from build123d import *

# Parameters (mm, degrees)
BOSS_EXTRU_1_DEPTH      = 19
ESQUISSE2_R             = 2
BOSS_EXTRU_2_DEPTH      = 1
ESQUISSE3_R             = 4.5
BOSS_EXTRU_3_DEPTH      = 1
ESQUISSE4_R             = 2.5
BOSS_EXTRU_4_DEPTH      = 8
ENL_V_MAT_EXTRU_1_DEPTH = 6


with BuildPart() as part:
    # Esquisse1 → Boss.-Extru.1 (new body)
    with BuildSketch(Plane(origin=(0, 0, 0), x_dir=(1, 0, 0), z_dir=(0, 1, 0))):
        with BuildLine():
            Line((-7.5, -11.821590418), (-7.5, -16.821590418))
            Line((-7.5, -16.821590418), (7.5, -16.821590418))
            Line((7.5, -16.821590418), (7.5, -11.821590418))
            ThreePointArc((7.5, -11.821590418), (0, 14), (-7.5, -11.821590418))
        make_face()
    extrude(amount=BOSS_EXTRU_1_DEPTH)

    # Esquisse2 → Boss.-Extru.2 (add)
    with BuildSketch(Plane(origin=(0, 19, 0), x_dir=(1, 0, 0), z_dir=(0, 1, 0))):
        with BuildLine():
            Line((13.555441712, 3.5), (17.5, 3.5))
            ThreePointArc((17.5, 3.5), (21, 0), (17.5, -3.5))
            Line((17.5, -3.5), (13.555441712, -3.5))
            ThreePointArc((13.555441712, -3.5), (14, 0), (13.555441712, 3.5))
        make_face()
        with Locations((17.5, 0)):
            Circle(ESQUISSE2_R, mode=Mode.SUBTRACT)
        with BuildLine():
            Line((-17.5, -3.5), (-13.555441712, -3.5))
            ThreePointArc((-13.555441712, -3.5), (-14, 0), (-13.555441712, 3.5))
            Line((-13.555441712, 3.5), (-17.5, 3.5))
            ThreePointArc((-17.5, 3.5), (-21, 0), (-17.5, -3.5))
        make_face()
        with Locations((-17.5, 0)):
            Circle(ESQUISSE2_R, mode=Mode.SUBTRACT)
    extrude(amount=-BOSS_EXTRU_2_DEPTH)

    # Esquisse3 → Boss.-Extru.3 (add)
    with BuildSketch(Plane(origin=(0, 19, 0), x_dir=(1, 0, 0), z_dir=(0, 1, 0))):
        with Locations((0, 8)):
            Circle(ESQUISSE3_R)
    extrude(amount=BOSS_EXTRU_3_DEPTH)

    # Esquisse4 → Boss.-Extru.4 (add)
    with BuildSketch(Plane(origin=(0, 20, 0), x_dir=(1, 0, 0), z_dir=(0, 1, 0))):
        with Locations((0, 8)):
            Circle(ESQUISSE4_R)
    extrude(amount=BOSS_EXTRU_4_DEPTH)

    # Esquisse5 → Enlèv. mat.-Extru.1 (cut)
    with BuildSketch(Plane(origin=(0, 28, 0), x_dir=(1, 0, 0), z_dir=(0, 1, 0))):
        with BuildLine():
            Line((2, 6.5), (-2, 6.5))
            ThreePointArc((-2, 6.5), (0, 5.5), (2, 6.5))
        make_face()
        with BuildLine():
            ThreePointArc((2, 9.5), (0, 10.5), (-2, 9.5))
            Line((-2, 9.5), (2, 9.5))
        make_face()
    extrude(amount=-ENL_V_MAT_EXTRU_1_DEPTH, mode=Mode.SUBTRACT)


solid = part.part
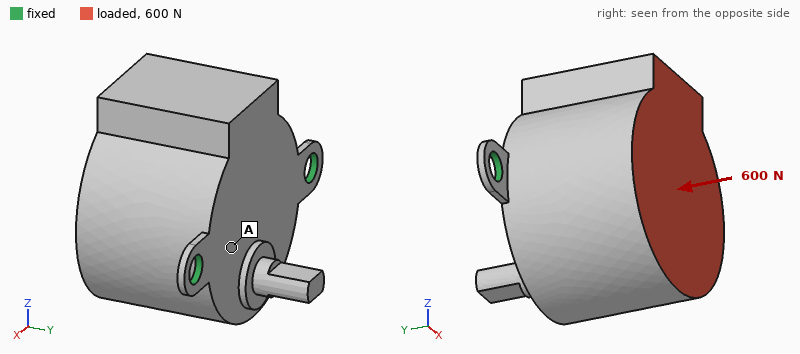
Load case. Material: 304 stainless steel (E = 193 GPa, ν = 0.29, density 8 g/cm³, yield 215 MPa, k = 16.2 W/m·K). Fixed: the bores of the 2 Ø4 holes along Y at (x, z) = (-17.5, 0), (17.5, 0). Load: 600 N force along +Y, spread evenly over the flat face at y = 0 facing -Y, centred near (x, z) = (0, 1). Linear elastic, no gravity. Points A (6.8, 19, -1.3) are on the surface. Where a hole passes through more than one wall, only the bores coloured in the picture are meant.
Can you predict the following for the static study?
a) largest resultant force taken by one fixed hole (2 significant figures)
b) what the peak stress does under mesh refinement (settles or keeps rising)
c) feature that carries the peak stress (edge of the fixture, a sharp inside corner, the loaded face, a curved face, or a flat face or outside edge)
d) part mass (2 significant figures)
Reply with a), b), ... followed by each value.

a) 350 N
b) keeps rising
c) edge of the fixture
d) 100 g
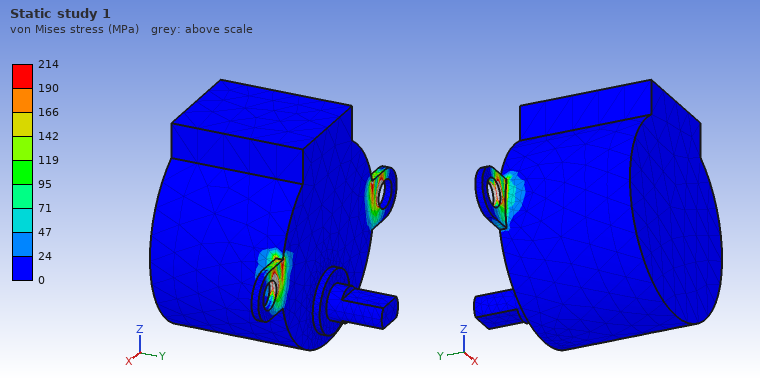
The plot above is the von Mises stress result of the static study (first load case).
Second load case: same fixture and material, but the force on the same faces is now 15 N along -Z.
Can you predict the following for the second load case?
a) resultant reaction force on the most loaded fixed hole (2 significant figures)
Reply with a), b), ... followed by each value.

a) 7.5 N
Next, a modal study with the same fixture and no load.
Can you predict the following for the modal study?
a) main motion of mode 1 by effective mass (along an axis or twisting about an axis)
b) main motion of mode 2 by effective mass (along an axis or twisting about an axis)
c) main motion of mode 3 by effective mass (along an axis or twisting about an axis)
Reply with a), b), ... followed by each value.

a) along Z
b) along Y
c) along X
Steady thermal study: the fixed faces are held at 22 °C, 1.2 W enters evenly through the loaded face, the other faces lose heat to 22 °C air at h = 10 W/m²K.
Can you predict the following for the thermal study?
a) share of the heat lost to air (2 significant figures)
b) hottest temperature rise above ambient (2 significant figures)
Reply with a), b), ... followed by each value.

a) 31 %
b) 15 K
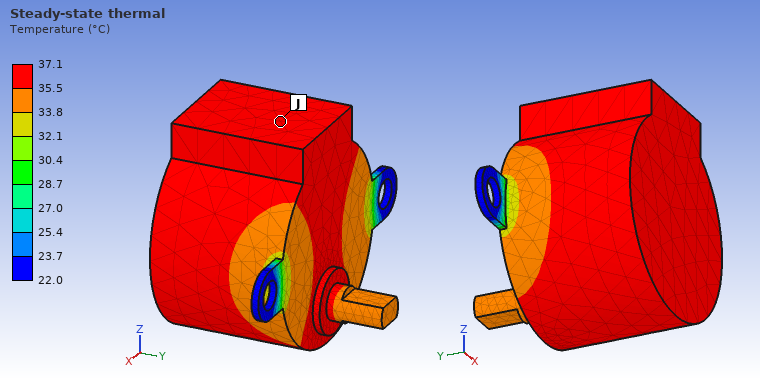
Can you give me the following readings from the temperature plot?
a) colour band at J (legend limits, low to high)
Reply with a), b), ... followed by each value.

a) 35.5 to 37.1 °C
